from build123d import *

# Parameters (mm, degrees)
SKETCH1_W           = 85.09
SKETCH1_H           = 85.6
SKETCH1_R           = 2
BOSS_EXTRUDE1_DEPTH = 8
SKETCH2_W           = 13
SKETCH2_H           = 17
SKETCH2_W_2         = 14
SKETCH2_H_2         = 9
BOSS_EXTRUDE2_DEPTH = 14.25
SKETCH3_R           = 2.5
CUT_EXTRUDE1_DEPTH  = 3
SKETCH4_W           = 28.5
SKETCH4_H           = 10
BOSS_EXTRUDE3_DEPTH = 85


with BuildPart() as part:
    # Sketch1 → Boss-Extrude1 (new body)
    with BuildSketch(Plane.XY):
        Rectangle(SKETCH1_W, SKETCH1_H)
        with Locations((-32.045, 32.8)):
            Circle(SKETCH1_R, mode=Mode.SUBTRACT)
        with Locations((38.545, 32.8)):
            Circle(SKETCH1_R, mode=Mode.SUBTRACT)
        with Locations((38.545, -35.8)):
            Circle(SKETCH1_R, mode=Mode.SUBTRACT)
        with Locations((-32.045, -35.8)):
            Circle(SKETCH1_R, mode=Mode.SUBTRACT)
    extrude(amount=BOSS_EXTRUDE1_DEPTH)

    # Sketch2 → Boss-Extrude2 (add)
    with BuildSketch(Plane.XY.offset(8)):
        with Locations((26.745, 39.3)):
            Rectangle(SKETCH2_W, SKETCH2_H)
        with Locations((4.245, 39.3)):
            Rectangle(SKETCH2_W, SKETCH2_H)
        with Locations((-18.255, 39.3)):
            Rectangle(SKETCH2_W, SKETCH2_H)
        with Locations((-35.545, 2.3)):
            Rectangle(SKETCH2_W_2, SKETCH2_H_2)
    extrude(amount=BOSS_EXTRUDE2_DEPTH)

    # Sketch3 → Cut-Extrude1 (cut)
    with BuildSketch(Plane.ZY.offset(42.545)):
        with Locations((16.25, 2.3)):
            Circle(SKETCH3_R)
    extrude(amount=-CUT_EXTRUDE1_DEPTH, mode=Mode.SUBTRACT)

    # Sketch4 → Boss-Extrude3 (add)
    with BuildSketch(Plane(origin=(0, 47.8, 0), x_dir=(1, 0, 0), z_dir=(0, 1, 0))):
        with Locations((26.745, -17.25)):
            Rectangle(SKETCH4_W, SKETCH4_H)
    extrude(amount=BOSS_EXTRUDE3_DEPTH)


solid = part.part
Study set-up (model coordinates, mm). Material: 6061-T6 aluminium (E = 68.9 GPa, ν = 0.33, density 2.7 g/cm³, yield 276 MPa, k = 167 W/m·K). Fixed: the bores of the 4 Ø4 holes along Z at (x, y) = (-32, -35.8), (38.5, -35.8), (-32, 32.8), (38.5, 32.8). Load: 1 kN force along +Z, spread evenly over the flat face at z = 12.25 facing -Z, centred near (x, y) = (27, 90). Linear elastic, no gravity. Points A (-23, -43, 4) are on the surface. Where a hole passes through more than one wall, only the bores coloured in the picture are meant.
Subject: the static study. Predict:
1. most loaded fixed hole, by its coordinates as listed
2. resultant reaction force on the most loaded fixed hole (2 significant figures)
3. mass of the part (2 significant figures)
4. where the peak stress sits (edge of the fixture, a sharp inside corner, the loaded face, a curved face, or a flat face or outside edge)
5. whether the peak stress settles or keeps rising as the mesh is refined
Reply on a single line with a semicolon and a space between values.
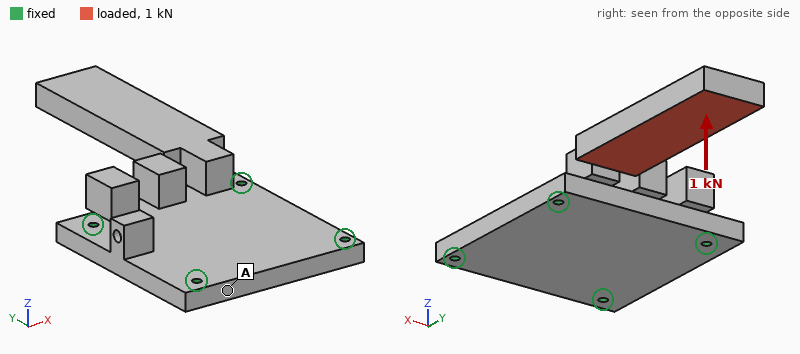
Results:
(38.5, 32.8); 1.2 kN; 250 g; edge of the fixture; keeps rising
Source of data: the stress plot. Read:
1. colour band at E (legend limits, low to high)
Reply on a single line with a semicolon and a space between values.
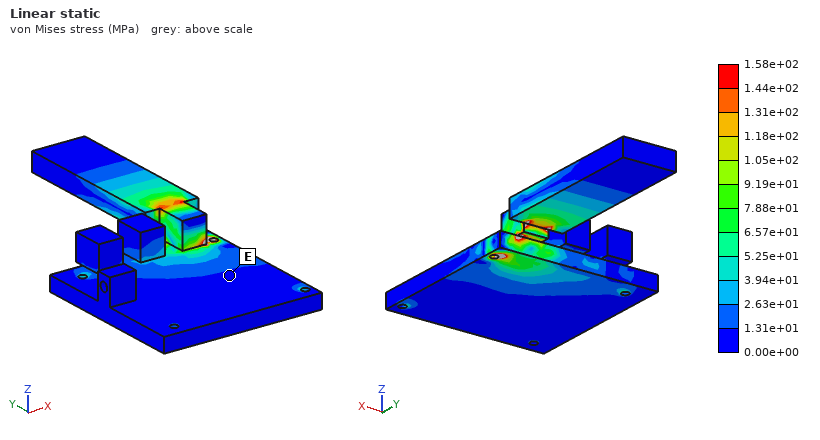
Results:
0.00e+00 to 1.31e+01 MPa
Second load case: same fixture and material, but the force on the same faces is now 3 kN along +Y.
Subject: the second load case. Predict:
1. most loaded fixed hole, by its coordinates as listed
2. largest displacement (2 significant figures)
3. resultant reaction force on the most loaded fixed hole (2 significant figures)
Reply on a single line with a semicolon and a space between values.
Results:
(38.5, 32.8); 88 µm; 1.8 kN
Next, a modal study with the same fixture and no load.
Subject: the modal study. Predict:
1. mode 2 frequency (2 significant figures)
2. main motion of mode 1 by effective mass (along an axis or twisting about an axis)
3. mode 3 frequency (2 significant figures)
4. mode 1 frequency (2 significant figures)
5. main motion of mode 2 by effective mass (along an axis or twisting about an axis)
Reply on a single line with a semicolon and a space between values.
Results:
880 Hz; along Z; 3300 Hz; 610 Hz; along X
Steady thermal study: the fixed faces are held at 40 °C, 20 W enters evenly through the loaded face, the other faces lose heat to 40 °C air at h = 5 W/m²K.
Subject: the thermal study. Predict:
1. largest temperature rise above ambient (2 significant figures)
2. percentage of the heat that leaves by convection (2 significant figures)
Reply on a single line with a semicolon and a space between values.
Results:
35 K; 4.3 %
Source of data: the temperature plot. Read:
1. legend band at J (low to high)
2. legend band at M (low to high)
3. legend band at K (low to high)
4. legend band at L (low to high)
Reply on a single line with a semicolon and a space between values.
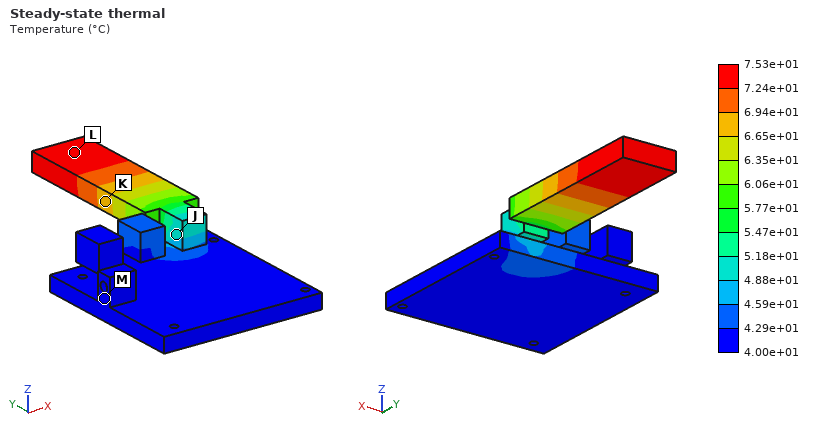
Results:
4.88e+01 to 5.18e+01 °C; 4.00e+01 to 4.29e+01 °C; 6.65e+01 to 6.94e+01 °C; 7.24e+01 to 7.53e+01 °C
